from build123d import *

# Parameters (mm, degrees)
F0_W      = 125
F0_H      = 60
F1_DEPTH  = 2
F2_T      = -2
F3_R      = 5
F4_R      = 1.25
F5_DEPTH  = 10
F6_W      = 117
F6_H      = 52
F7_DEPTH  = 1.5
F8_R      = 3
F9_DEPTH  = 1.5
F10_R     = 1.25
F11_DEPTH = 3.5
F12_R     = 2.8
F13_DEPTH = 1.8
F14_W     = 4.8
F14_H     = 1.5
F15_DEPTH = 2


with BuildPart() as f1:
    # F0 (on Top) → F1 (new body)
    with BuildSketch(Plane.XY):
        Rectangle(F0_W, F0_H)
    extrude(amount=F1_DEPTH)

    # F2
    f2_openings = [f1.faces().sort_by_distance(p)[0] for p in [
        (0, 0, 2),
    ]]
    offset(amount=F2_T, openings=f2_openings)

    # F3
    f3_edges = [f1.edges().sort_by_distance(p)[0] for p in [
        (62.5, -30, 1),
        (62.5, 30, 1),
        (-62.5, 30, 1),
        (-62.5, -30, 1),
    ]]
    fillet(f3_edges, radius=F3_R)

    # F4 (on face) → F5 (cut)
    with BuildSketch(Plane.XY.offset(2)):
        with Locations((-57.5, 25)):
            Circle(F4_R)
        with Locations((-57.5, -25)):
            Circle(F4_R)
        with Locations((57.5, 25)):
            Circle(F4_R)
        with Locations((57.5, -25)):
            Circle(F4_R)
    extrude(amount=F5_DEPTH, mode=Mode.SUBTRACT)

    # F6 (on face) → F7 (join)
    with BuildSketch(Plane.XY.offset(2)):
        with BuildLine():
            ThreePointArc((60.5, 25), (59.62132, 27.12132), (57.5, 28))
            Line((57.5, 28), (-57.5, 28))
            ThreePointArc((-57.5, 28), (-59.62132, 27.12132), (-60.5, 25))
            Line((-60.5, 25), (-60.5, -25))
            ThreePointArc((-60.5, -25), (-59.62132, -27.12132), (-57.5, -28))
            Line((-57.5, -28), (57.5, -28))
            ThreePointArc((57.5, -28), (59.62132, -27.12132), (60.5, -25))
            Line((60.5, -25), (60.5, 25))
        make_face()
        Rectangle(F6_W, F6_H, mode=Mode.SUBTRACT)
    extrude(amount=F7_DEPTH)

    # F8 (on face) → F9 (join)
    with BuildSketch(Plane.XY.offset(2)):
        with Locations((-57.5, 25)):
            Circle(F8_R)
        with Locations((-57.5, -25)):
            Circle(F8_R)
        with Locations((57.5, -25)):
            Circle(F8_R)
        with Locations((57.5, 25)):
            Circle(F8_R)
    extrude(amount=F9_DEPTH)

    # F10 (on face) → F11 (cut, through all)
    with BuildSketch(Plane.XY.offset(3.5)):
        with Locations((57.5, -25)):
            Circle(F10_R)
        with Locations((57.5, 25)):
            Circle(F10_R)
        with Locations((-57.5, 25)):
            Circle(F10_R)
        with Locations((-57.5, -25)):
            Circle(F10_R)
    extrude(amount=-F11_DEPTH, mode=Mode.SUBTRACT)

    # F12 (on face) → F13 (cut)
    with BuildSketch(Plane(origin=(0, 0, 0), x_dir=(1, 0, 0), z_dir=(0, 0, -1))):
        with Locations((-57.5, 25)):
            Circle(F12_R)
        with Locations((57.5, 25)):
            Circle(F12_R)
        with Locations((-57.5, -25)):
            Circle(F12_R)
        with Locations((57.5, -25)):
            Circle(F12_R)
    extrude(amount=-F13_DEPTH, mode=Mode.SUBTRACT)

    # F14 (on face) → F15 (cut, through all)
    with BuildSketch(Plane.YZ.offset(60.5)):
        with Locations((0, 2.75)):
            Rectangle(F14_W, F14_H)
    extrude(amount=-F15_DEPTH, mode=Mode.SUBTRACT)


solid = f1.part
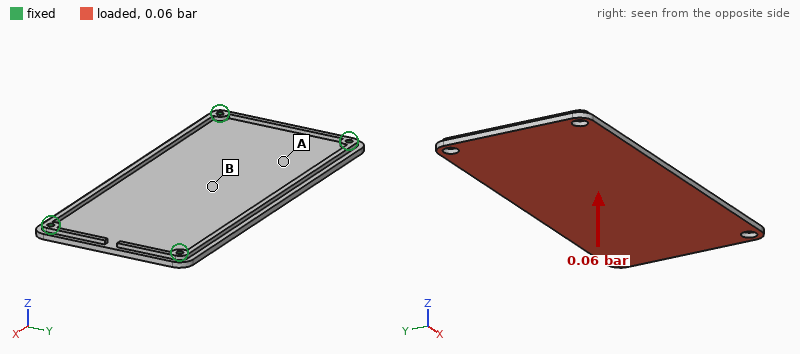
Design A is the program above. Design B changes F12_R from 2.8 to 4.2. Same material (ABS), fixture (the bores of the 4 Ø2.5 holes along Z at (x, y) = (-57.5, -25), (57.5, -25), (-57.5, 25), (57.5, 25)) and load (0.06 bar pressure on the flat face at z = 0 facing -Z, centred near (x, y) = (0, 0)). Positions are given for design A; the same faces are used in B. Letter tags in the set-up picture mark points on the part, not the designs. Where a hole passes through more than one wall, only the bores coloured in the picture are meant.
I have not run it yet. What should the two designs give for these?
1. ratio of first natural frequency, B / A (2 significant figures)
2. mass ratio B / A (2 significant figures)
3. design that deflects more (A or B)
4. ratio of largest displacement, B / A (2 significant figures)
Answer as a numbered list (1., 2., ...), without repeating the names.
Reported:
1. 0.94
2. 0.99
3. B
4. 1.1
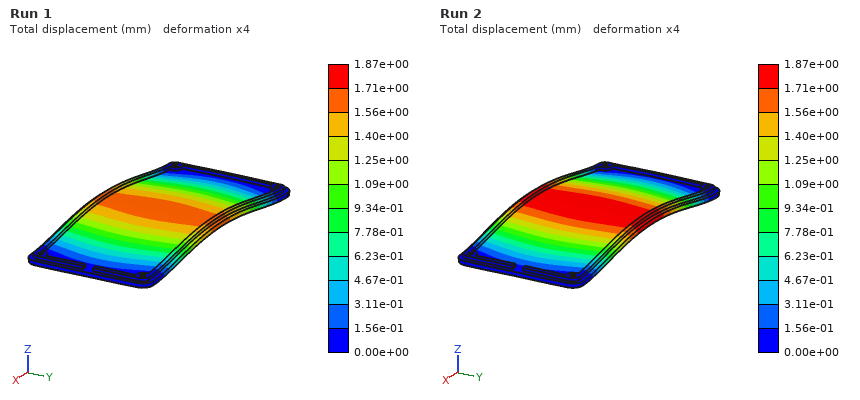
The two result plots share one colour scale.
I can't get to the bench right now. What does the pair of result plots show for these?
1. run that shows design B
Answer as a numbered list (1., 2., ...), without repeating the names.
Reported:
1. Run 2
